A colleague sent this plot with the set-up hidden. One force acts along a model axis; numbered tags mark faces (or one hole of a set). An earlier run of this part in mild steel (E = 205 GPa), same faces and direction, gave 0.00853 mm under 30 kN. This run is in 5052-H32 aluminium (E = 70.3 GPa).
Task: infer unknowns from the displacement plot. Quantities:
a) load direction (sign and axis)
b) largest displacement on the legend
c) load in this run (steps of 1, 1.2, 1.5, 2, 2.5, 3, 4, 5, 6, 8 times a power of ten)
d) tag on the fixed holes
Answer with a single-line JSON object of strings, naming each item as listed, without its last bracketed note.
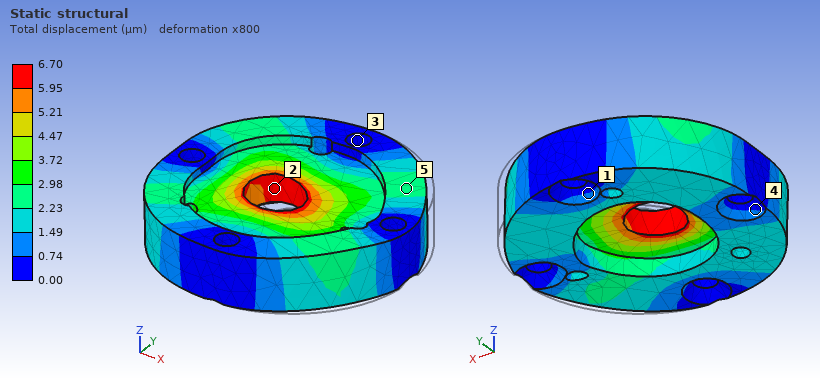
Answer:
{"load direction": "-X", "largest displacement on the legend": "6.70 µm", "load in this run": "8 kN", "tag on the fixed holes": "3"}
